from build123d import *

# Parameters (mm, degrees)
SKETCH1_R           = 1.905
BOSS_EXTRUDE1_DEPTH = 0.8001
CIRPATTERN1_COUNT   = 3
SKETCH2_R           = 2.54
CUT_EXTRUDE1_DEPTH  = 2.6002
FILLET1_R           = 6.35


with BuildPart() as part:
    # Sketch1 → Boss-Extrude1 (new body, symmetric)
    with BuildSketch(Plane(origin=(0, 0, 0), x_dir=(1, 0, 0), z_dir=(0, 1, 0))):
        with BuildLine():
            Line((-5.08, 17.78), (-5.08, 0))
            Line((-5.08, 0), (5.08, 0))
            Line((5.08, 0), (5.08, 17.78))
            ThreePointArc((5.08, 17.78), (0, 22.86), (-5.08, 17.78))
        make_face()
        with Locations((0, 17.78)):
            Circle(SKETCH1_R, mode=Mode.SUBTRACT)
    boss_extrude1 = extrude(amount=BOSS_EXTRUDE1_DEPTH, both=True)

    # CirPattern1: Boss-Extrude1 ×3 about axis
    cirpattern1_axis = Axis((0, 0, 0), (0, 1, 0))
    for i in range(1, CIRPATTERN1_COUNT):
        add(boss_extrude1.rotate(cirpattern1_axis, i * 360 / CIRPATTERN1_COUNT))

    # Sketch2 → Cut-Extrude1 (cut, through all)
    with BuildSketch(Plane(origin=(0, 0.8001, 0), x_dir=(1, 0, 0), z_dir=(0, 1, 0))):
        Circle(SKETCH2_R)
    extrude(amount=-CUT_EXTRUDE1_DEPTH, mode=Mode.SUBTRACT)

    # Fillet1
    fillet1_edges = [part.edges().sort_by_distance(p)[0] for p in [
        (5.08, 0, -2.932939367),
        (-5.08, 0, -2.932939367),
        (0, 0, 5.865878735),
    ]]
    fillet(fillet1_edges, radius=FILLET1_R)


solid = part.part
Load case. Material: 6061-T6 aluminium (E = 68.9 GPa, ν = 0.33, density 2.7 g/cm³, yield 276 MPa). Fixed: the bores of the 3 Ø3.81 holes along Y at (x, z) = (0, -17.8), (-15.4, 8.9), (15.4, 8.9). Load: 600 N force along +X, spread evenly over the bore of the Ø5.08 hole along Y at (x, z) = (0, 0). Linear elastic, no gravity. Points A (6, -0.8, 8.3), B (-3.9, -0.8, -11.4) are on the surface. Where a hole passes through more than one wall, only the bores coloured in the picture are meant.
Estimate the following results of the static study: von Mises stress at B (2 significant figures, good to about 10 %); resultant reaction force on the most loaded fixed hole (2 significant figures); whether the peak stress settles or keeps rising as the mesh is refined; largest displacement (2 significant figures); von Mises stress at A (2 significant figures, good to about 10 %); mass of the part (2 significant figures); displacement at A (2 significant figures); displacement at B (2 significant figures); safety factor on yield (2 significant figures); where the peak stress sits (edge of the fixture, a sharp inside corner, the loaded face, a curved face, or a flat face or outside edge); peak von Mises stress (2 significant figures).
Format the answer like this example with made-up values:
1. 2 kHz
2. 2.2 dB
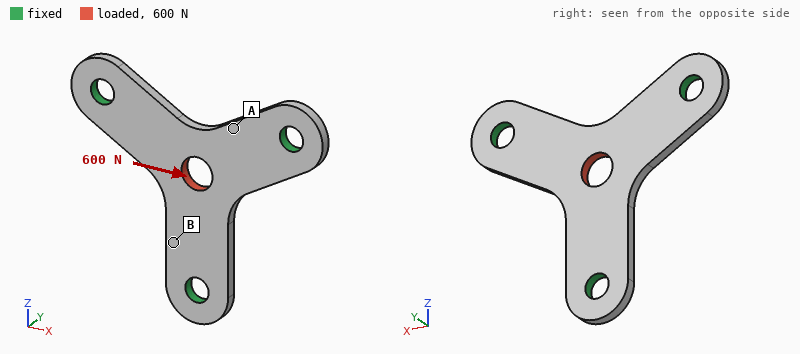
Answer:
1. 7.2 MPa
2. 300 N
3. settles
4. 8.5 µm
5. 18 MPa
6. 2.5 g
7. 2.1 µm
8. 3.1 µm
9. 4.7
10. the loaded face
11. 59 MPa
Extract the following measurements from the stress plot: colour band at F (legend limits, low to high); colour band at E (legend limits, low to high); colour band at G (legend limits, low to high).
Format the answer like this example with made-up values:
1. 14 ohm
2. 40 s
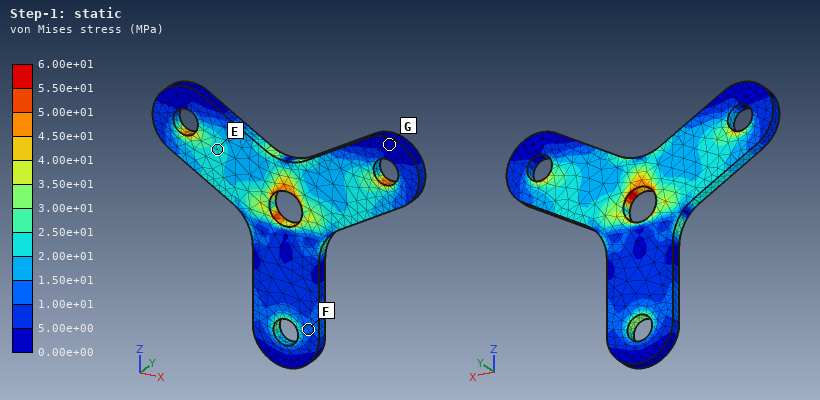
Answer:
1. 1.00e+01 to 1.50e+01 MPa
2. 2.00e+01 to 2.50e+01 MPa
3. 0.00e+00 to 5.00e+00 MPa
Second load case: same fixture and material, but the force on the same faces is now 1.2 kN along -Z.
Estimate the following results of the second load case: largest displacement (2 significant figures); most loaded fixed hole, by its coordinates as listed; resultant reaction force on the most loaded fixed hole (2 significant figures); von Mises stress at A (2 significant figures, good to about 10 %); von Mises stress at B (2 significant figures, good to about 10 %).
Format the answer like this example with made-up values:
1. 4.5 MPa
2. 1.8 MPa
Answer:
1. 17 µm
2. (0, -17.8)
3. 700 N
4. 29 MPa
5. 41 MPa
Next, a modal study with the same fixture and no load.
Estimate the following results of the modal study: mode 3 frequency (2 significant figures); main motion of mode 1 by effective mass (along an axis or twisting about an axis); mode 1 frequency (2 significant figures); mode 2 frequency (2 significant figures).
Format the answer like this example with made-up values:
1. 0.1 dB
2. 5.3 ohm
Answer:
1. 19 kHz
2. along Y
3. 9200 Hz
4. 19 kHz
